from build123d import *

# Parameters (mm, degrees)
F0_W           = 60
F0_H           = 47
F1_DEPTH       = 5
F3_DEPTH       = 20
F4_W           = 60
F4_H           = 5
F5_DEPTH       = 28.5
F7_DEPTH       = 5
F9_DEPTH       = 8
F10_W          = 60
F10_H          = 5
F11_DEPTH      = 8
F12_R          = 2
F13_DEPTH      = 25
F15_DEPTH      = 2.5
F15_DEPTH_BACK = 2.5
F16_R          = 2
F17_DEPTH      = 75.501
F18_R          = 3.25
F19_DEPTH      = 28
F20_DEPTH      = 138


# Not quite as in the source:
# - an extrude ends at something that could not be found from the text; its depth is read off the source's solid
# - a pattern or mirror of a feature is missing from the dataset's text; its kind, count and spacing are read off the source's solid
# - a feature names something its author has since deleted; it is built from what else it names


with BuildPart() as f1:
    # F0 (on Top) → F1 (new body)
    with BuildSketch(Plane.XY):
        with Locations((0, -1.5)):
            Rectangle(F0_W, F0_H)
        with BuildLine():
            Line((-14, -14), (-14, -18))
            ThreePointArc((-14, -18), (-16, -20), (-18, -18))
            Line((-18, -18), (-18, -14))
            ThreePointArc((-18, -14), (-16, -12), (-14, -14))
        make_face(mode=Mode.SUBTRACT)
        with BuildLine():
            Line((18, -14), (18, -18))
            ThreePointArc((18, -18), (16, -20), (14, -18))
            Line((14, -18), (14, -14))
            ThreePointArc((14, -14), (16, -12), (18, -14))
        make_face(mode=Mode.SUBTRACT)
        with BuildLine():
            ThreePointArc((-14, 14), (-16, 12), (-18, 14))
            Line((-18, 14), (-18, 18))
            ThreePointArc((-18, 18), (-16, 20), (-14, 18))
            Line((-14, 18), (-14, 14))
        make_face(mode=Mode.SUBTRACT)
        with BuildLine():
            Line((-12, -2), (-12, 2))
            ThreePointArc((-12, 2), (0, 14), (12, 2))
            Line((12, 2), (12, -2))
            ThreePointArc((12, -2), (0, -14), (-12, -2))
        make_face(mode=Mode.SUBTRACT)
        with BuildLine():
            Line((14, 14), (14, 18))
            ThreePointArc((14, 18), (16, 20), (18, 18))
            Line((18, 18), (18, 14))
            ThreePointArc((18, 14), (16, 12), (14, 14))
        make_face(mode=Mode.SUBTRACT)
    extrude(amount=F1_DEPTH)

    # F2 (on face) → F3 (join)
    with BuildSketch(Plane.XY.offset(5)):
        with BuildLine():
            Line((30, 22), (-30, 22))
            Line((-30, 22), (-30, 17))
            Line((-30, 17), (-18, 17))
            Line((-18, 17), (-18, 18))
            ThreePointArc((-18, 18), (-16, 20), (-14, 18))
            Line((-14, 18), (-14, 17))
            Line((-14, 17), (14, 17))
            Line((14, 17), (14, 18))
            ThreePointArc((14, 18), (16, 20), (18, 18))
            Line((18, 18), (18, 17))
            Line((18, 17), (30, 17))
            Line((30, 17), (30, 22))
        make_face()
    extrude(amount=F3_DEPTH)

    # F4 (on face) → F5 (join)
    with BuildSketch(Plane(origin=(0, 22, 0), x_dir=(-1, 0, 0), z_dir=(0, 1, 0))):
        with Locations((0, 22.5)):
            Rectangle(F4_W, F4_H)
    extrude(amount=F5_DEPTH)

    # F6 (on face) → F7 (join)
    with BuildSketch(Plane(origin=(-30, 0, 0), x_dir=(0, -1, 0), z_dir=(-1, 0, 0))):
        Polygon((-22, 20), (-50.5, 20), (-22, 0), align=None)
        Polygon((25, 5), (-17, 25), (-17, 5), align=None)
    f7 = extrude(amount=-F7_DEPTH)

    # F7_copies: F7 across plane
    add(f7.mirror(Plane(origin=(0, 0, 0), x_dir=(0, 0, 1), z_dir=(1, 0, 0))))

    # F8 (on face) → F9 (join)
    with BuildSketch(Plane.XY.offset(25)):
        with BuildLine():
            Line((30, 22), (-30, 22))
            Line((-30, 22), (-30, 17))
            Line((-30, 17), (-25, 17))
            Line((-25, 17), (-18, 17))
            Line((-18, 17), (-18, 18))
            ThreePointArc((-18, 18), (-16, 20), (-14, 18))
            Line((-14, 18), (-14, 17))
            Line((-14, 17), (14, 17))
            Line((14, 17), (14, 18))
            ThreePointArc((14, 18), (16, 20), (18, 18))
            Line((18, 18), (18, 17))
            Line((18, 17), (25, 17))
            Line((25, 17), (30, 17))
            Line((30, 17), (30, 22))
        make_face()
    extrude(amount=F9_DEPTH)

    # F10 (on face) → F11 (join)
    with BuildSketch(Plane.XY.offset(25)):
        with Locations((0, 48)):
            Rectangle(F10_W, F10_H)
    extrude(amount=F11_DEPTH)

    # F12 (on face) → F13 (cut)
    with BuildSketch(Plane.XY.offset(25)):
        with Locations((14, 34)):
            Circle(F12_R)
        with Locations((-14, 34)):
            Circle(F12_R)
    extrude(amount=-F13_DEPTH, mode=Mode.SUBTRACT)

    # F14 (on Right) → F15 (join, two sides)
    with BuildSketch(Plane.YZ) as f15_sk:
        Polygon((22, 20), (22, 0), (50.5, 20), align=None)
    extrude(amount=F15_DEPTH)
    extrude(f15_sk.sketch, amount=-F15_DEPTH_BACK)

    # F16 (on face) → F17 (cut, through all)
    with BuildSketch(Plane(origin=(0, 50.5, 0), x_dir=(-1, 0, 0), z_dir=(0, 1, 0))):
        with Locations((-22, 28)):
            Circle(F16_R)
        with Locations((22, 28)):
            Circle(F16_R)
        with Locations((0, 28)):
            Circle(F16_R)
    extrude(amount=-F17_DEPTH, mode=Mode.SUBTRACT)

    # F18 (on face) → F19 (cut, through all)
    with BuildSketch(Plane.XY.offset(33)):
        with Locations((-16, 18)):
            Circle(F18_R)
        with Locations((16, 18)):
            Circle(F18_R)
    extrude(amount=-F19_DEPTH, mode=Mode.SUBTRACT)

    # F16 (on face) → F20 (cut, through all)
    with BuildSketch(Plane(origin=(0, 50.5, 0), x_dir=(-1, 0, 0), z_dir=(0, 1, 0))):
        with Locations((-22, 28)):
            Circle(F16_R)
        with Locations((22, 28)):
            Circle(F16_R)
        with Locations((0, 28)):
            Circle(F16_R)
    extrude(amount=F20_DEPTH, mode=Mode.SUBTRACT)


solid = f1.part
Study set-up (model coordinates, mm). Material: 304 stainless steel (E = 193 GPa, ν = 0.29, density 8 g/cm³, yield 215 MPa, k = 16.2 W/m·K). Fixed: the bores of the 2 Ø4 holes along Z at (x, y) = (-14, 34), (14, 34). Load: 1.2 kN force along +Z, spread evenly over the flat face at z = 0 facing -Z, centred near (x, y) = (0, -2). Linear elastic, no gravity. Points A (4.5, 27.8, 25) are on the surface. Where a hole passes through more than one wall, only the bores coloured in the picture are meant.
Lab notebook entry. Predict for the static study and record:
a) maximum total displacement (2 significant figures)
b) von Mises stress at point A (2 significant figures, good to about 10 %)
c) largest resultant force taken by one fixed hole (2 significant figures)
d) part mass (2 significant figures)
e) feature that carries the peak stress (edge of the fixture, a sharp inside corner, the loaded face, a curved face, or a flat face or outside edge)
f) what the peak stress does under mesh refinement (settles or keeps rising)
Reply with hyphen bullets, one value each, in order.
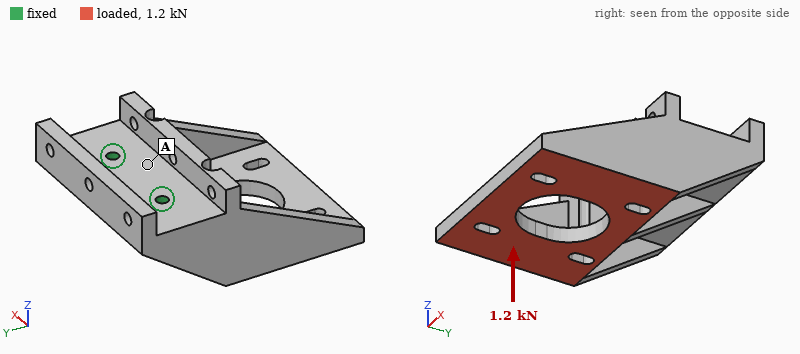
- 0.14 mm
- 31 MPa
- 620 N
- 290 g
- edge of the fixture
- keeps rising
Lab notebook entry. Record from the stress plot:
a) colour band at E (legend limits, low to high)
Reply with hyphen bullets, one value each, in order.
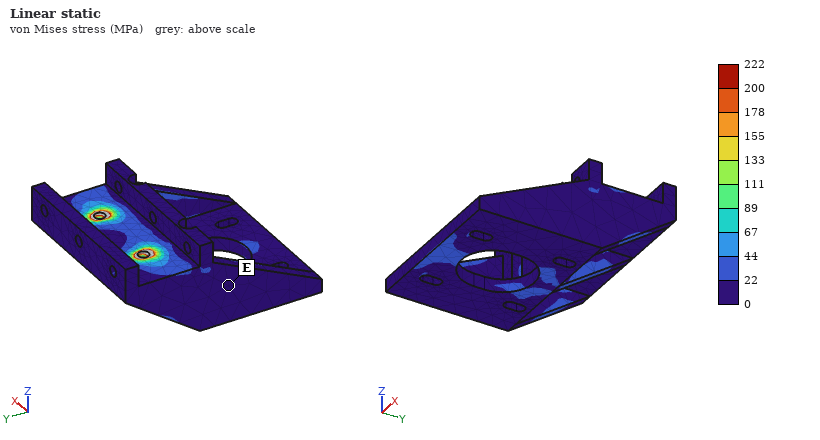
- 0 to 22 MPa
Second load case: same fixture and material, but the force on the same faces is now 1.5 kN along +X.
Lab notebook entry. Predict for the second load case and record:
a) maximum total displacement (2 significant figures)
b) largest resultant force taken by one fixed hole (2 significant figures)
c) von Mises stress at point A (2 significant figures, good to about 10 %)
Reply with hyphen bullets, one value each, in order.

- 25 µm
- 2.2 kN
- 9.6 MPa
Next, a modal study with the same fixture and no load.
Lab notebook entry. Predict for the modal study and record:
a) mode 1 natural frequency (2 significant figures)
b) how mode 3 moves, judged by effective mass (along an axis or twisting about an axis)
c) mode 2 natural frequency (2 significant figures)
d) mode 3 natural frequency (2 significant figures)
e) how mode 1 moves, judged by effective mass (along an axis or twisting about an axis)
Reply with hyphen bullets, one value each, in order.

- 1500 Hz
- along X
- 2500 Hz
- 4100 Hz
- along Z
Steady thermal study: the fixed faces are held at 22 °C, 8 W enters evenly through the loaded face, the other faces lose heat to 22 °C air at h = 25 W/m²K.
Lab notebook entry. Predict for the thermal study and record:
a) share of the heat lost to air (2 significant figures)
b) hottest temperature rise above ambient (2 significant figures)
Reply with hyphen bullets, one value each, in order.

- 66 %
- 38 K
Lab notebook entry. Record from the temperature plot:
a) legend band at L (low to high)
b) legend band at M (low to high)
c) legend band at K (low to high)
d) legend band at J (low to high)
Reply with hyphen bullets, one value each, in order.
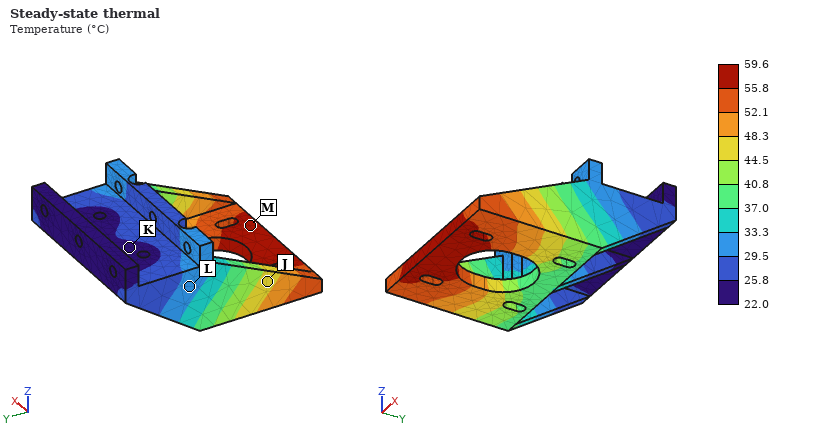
- 29.5 to 33.3 °C
- 55.8 to 59.6 °C
- 22.0 to 25.8 °C
- 44.5 to 48.3 °C
